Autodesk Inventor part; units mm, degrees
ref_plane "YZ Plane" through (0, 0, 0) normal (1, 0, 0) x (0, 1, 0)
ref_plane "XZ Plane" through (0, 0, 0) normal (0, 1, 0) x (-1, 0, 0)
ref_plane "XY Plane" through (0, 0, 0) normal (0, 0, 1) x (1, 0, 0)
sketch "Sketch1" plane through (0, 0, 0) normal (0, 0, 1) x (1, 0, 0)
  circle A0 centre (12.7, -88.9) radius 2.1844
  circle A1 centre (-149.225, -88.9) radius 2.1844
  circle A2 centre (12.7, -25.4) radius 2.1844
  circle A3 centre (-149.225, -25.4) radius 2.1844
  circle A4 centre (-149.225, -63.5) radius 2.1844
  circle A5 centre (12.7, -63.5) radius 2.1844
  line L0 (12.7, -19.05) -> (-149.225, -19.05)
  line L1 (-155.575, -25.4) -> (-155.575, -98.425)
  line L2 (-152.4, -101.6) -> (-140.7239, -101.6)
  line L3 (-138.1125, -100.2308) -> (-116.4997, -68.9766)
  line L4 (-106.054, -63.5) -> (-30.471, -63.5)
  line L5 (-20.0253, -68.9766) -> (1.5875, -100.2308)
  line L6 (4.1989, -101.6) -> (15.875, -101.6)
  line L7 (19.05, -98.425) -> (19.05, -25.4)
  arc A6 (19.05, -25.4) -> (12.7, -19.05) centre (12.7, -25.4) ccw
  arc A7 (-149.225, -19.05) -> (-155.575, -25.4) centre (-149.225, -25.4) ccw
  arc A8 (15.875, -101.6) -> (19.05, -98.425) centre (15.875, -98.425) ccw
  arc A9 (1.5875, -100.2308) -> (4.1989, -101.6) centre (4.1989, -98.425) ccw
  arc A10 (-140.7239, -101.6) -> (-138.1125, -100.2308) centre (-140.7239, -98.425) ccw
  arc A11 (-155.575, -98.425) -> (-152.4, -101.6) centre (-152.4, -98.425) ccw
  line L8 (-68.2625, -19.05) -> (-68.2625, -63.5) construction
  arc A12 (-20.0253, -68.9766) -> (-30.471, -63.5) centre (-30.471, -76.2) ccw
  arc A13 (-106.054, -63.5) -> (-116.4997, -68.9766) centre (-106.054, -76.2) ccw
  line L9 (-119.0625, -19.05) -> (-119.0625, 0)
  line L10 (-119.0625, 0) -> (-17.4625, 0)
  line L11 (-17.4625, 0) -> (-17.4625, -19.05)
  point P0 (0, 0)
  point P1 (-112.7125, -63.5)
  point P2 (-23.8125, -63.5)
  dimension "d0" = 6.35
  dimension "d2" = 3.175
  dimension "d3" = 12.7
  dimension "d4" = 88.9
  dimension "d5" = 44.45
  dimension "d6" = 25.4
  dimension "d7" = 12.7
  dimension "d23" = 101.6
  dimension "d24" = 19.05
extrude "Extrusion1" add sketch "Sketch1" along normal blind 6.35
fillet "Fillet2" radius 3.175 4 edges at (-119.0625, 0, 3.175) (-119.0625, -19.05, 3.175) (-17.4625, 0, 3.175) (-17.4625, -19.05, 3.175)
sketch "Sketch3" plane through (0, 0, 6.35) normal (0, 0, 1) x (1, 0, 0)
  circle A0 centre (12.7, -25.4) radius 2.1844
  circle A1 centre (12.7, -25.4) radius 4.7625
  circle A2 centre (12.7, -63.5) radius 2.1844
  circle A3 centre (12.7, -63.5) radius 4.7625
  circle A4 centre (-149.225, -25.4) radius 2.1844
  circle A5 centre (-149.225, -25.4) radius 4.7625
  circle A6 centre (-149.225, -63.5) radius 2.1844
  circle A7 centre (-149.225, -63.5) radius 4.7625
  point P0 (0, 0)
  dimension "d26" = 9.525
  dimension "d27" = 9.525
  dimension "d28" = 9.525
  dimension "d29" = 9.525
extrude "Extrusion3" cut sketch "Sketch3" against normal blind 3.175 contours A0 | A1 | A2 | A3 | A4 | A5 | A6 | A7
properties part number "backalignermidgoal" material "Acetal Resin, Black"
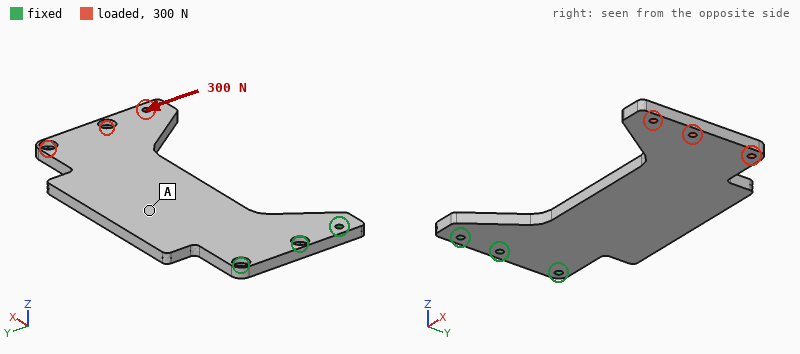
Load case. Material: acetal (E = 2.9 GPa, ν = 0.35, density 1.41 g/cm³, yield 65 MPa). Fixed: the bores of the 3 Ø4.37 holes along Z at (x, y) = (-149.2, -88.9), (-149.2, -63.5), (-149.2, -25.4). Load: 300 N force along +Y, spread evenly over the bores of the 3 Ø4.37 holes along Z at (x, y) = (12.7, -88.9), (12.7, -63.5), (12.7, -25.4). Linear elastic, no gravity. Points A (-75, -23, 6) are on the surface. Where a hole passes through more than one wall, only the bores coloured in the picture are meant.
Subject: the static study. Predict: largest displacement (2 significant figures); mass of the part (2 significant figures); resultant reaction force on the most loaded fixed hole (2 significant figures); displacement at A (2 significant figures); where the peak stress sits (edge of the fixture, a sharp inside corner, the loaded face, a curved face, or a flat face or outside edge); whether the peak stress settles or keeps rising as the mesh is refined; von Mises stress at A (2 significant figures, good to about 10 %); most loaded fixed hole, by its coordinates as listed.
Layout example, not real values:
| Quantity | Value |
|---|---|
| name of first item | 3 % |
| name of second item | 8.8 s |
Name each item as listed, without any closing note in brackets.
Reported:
| Quantity | Value |
|---|---|
| largest displacement | 2.3 mm |
| mass of the part | 110 g |
| resultant reaction force on the most loaded fixed hole | 890 N |
| displacement at A | 0.80 mm |
| where the peak stress sits | edge of the fixture |
| whether the peak stress settles or keeps rising as the mesh is refined | keeps rising |
| von Mises stress at A | 2.7 MPa |
| most loaded fixed hole, by its coordinates as listed | (-149.2, -25.4) |
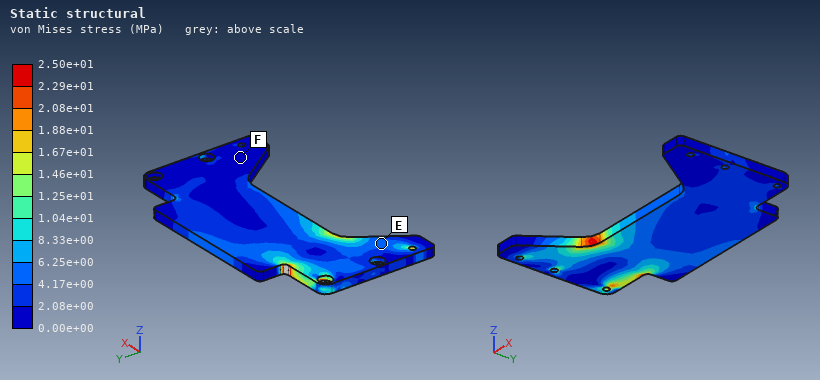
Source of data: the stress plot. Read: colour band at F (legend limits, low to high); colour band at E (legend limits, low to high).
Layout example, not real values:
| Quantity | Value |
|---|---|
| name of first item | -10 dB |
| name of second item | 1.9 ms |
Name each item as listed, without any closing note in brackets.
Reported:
| Quantity | Value |
|---|---|
| colour band at F | 0.00e+00 to 2.08e+00 MPa |
| colour band at E | 4.17e+00 to 6.25e+00 MPa |
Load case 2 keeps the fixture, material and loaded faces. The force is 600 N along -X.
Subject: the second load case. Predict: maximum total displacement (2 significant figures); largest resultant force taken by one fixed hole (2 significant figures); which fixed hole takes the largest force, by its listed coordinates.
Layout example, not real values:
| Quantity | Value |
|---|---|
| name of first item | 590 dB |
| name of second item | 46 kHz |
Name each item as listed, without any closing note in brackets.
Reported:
| Quantity | Value |
|---|---|
| maximum total displacement | 2.0 mm |
| largest resultant force taken by one fixed hole | 330 N |
| which fixed hole takes the largest force, by its listed coordinates | (-149.2, -63.5) |
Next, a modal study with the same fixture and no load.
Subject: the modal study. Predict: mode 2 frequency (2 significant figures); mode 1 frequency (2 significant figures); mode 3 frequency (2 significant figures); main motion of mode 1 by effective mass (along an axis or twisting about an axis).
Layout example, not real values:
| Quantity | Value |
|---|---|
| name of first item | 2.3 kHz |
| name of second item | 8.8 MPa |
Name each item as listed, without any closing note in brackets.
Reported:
| Quantity | Value |
|---|---|
| mode 2 frequency | 170 Hz |
| mode 1 frequency | 42 Hz |
| mode 3 frequency | 340 Hz |
| main motion of mode 1 by effective mass | along Z |
